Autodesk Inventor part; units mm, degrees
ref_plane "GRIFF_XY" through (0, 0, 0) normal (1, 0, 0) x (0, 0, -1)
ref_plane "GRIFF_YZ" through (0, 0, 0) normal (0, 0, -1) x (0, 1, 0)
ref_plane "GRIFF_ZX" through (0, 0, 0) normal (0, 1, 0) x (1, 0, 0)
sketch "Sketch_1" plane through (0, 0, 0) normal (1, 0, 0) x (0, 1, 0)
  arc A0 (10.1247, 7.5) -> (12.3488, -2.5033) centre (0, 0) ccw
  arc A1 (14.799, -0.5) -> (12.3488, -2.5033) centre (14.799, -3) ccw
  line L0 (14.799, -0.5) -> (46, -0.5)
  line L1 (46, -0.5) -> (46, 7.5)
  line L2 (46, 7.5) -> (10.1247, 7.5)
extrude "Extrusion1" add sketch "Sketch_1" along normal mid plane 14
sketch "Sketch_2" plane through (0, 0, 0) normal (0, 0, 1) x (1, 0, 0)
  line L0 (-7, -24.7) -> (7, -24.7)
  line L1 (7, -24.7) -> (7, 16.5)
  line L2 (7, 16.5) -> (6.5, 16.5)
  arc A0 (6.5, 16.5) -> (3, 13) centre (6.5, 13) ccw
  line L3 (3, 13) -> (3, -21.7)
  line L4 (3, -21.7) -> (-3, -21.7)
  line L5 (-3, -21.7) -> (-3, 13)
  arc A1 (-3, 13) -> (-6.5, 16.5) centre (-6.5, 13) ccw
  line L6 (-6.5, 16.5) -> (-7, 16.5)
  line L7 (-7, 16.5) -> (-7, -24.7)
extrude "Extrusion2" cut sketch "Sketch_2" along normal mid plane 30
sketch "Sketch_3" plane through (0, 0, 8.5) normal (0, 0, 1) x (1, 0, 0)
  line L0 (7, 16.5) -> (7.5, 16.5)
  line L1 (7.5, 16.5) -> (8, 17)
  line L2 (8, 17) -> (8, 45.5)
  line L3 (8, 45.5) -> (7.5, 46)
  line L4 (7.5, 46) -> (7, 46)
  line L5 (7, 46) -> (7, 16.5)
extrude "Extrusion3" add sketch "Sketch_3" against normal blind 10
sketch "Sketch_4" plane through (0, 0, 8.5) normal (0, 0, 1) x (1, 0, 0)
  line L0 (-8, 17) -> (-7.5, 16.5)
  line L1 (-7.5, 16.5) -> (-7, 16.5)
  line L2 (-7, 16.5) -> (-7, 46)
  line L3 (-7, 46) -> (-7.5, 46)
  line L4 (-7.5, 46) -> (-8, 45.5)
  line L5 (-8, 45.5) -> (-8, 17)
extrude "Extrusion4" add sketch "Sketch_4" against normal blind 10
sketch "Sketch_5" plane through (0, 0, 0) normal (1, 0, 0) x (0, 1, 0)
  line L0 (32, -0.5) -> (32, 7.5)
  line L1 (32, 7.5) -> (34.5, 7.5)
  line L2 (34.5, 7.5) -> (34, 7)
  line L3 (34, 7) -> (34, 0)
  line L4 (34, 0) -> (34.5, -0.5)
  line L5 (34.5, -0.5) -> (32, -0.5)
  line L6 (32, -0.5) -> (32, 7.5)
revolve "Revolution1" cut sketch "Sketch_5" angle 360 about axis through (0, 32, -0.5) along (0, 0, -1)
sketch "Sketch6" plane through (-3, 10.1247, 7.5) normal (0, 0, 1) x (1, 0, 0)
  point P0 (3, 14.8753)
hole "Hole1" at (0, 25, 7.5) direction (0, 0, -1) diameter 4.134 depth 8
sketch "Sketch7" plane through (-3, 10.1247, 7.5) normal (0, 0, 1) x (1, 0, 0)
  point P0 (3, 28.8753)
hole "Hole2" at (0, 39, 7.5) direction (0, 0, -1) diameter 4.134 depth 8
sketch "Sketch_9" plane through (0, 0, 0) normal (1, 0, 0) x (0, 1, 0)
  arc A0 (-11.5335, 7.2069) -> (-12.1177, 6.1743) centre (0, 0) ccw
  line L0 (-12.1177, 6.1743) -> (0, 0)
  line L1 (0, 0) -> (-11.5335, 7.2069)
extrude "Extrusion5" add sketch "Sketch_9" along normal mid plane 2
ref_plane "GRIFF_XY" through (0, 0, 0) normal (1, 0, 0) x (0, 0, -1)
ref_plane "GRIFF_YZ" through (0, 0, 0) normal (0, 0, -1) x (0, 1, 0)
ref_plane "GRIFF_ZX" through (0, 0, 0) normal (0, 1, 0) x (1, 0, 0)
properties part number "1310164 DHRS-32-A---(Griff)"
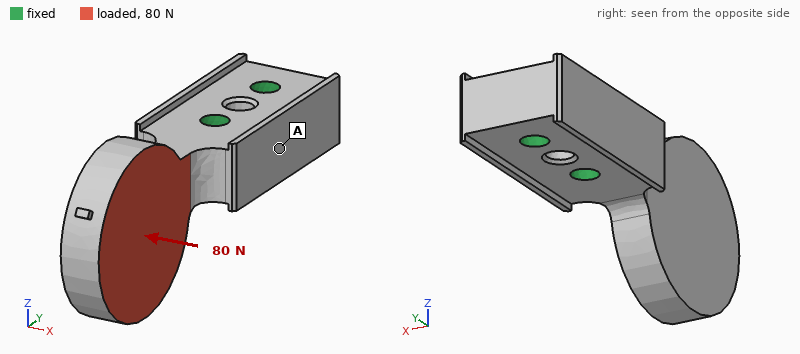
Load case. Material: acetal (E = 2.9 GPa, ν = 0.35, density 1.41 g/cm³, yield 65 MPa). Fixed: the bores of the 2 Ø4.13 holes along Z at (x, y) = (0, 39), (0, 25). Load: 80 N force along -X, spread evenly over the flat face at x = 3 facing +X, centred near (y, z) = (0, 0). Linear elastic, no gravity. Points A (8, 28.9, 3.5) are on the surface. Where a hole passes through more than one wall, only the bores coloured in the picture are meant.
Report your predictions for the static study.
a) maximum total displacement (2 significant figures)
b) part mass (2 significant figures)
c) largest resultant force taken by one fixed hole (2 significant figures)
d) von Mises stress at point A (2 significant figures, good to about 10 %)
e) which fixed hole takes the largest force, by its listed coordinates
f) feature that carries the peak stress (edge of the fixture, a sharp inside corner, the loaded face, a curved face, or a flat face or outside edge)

0.64 mm
9.6 g
150 N
3.3 MPa
(0, 25)
a curved face
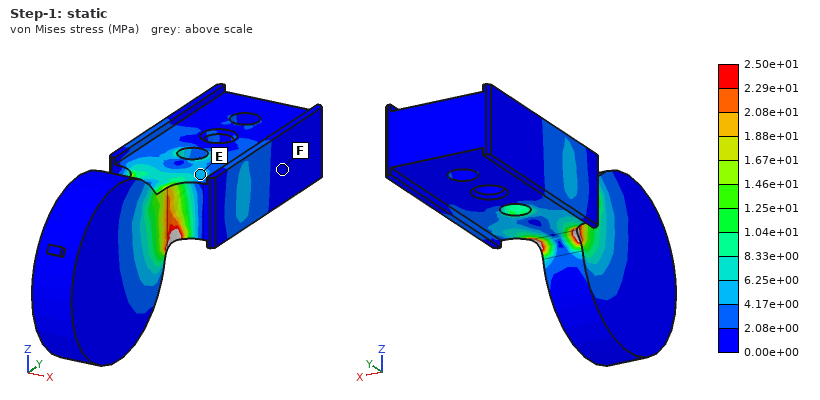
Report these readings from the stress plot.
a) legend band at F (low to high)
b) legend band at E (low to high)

0.00e+00 to 2.08e+00 MPa
4.17e+00 to 6.25e+00 MPa
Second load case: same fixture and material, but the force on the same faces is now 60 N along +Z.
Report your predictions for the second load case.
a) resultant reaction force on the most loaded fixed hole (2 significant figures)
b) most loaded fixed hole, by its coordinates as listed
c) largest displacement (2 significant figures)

83 N
(0, 25)
0.43 mm
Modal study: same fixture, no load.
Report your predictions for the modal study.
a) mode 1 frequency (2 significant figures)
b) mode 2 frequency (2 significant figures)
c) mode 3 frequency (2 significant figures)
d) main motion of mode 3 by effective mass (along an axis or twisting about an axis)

1100 Hz
1100 Hz
2400 Hz
twisting about Y
